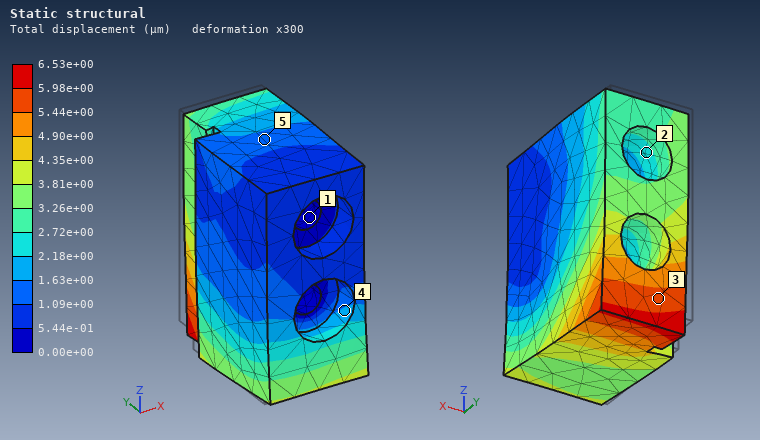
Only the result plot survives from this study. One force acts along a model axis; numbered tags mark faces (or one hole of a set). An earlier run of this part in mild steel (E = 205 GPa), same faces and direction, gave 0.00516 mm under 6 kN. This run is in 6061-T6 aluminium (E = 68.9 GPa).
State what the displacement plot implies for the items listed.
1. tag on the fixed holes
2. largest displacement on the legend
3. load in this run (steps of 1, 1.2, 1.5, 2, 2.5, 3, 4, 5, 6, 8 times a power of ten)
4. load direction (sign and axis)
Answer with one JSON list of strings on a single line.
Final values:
["1", "6.53e+00 µm", "2.5 kN", "-Y"]
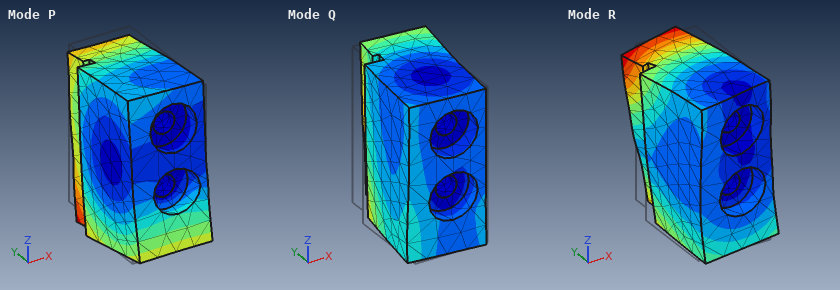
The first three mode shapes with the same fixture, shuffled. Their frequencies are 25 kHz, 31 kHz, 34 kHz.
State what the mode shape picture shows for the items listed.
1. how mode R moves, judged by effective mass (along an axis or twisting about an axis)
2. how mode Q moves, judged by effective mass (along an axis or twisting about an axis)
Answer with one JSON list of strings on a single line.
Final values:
["twisting about Y", "along X"]
